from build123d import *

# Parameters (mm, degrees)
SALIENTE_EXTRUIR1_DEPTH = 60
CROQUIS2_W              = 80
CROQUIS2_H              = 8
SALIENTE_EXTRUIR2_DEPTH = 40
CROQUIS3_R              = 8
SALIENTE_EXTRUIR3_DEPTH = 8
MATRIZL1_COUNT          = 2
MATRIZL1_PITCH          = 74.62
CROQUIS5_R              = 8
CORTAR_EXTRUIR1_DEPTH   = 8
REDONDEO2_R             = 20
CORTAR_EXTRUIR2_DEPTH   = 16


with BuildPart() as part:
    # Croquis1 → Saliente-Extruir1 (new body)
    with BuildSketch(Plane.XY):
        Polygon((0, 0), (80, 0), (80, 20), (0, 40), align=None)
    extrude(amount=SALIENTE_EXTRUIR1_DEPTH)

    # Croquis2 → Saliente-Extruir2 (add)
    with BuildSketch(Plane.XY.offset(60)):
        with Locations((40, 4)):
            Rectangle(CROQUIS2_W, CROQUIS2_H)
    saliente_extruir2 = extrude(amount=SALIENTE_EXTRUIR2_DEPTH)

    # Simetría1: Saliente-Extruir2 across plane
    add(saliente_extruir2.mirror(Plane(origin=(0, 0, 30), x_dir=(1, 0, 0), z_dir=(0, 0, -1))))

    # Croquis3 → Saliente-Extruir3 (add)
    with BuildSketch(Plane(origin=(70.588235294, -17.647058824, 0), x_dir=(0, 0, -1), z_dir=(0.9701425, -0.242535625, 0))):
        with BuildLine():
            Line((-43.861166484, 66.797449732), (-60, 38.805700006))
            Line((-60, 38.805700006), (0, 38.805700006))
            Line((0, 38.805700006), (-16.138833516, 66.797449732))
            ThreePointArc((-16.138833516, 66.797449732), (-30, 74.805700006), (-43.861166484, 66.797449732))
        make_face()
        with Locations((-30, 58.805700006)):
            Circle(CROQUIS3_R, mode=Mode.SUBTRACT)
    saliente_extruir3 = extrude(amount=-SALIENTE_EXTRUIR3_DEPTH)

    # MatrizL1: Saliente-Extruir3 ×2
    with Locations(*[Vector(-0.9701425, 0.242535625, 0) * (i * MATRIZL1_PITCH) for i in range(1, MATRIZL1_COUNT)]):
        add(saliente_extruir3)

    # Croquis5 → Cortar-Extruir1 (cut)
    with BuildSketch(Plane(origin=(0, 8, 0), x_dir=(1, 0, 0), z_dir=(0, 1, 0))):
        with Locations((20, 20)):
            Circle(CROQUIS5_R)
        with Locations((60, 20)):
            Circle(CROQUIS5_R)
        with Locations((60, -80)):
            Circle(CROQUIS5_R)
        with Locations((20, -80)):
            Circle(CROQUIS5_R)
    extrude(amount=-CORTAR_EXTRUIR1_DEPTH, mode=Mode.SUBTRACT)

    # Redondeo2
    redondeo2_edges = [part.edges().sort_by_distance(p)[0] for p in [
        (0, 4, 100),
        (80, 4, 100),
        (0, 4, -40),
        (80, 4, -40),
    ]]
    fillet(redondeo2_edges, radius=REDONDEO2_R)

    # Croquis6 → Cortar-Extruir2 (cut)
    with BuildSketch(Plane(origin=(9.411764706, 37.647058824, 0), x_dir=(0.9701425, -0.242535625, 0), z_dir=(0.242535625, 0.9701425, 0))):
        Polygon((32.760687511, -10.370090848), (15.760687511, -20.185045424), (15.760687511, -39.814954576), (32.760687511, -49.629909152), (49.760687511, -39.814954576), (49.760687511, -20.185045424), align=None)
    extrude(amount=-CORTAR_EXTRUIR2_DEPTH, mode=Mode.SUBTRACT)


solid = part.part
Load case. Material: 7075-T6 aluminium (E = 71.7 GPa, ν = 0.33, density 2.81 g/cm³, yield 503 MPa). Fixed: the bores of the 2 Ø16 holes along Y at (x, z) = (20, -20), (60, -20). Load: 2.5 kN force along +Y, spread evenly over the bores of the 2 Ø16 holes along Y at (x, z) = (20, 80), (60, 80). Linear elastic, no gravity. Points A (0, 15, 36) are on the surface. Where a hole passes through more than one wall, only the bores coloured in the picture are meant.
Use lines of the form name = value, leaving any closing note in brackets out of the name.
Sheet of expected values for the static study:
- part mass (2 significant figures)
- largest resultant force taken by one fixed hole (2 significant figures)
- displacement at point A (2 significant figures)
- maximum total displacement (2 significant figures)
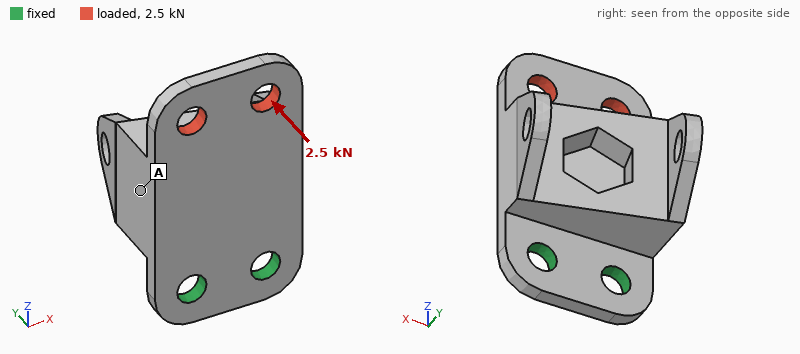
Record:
part mass = 530 g
largest resultant force taken by one fixed hole = 1.3 kN
displacement at point A = 0.67 mm
maximum total displacement = 1.8 mm
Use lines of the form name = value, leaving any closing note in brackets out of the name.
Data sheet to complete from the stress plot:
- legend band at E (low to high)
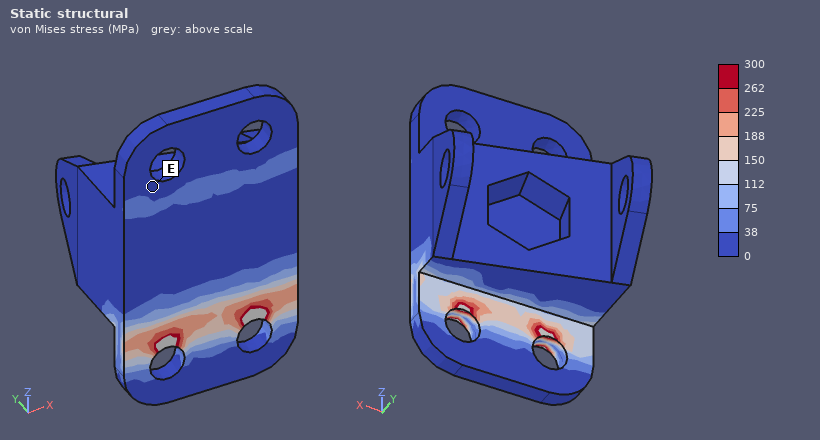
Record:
legend band at E = 0 to 38 MPa
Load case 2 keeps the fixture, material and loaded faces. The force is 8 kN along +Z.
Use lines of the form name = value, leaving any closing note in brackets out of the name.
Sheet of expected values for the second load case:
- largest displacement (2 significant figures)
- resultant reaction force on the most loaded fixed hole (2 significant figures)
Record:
largest displacement = 48 µm
resultant reaction force on the most loaded fixed hole = 4.0 kN
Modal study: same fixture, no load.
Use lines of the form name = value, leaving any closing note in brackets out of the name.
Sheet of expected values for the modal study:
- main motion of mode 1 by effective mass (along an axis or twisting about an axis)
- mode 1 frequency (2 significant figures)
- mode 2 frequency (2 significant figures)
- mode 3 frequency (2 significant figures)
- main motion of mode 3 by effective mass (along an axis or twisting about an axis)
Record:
main motion of mode 1 by effective mass = along Y
mode 1 frequency = 520 Hz
mode 2 frequency = 2200 Hz
mode 3 frequency = 2900 Hz
main motion of mode 3 by effective mass = along X
